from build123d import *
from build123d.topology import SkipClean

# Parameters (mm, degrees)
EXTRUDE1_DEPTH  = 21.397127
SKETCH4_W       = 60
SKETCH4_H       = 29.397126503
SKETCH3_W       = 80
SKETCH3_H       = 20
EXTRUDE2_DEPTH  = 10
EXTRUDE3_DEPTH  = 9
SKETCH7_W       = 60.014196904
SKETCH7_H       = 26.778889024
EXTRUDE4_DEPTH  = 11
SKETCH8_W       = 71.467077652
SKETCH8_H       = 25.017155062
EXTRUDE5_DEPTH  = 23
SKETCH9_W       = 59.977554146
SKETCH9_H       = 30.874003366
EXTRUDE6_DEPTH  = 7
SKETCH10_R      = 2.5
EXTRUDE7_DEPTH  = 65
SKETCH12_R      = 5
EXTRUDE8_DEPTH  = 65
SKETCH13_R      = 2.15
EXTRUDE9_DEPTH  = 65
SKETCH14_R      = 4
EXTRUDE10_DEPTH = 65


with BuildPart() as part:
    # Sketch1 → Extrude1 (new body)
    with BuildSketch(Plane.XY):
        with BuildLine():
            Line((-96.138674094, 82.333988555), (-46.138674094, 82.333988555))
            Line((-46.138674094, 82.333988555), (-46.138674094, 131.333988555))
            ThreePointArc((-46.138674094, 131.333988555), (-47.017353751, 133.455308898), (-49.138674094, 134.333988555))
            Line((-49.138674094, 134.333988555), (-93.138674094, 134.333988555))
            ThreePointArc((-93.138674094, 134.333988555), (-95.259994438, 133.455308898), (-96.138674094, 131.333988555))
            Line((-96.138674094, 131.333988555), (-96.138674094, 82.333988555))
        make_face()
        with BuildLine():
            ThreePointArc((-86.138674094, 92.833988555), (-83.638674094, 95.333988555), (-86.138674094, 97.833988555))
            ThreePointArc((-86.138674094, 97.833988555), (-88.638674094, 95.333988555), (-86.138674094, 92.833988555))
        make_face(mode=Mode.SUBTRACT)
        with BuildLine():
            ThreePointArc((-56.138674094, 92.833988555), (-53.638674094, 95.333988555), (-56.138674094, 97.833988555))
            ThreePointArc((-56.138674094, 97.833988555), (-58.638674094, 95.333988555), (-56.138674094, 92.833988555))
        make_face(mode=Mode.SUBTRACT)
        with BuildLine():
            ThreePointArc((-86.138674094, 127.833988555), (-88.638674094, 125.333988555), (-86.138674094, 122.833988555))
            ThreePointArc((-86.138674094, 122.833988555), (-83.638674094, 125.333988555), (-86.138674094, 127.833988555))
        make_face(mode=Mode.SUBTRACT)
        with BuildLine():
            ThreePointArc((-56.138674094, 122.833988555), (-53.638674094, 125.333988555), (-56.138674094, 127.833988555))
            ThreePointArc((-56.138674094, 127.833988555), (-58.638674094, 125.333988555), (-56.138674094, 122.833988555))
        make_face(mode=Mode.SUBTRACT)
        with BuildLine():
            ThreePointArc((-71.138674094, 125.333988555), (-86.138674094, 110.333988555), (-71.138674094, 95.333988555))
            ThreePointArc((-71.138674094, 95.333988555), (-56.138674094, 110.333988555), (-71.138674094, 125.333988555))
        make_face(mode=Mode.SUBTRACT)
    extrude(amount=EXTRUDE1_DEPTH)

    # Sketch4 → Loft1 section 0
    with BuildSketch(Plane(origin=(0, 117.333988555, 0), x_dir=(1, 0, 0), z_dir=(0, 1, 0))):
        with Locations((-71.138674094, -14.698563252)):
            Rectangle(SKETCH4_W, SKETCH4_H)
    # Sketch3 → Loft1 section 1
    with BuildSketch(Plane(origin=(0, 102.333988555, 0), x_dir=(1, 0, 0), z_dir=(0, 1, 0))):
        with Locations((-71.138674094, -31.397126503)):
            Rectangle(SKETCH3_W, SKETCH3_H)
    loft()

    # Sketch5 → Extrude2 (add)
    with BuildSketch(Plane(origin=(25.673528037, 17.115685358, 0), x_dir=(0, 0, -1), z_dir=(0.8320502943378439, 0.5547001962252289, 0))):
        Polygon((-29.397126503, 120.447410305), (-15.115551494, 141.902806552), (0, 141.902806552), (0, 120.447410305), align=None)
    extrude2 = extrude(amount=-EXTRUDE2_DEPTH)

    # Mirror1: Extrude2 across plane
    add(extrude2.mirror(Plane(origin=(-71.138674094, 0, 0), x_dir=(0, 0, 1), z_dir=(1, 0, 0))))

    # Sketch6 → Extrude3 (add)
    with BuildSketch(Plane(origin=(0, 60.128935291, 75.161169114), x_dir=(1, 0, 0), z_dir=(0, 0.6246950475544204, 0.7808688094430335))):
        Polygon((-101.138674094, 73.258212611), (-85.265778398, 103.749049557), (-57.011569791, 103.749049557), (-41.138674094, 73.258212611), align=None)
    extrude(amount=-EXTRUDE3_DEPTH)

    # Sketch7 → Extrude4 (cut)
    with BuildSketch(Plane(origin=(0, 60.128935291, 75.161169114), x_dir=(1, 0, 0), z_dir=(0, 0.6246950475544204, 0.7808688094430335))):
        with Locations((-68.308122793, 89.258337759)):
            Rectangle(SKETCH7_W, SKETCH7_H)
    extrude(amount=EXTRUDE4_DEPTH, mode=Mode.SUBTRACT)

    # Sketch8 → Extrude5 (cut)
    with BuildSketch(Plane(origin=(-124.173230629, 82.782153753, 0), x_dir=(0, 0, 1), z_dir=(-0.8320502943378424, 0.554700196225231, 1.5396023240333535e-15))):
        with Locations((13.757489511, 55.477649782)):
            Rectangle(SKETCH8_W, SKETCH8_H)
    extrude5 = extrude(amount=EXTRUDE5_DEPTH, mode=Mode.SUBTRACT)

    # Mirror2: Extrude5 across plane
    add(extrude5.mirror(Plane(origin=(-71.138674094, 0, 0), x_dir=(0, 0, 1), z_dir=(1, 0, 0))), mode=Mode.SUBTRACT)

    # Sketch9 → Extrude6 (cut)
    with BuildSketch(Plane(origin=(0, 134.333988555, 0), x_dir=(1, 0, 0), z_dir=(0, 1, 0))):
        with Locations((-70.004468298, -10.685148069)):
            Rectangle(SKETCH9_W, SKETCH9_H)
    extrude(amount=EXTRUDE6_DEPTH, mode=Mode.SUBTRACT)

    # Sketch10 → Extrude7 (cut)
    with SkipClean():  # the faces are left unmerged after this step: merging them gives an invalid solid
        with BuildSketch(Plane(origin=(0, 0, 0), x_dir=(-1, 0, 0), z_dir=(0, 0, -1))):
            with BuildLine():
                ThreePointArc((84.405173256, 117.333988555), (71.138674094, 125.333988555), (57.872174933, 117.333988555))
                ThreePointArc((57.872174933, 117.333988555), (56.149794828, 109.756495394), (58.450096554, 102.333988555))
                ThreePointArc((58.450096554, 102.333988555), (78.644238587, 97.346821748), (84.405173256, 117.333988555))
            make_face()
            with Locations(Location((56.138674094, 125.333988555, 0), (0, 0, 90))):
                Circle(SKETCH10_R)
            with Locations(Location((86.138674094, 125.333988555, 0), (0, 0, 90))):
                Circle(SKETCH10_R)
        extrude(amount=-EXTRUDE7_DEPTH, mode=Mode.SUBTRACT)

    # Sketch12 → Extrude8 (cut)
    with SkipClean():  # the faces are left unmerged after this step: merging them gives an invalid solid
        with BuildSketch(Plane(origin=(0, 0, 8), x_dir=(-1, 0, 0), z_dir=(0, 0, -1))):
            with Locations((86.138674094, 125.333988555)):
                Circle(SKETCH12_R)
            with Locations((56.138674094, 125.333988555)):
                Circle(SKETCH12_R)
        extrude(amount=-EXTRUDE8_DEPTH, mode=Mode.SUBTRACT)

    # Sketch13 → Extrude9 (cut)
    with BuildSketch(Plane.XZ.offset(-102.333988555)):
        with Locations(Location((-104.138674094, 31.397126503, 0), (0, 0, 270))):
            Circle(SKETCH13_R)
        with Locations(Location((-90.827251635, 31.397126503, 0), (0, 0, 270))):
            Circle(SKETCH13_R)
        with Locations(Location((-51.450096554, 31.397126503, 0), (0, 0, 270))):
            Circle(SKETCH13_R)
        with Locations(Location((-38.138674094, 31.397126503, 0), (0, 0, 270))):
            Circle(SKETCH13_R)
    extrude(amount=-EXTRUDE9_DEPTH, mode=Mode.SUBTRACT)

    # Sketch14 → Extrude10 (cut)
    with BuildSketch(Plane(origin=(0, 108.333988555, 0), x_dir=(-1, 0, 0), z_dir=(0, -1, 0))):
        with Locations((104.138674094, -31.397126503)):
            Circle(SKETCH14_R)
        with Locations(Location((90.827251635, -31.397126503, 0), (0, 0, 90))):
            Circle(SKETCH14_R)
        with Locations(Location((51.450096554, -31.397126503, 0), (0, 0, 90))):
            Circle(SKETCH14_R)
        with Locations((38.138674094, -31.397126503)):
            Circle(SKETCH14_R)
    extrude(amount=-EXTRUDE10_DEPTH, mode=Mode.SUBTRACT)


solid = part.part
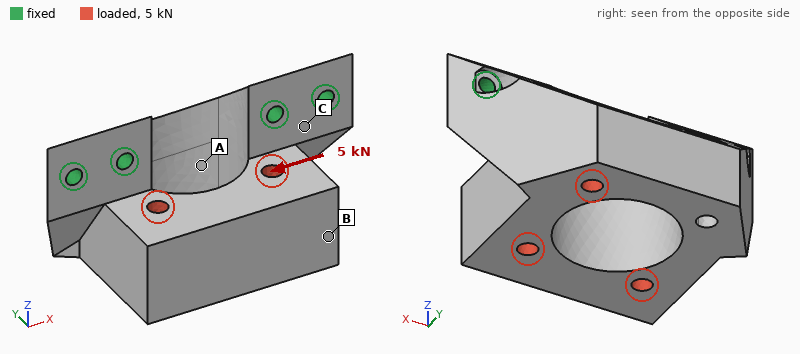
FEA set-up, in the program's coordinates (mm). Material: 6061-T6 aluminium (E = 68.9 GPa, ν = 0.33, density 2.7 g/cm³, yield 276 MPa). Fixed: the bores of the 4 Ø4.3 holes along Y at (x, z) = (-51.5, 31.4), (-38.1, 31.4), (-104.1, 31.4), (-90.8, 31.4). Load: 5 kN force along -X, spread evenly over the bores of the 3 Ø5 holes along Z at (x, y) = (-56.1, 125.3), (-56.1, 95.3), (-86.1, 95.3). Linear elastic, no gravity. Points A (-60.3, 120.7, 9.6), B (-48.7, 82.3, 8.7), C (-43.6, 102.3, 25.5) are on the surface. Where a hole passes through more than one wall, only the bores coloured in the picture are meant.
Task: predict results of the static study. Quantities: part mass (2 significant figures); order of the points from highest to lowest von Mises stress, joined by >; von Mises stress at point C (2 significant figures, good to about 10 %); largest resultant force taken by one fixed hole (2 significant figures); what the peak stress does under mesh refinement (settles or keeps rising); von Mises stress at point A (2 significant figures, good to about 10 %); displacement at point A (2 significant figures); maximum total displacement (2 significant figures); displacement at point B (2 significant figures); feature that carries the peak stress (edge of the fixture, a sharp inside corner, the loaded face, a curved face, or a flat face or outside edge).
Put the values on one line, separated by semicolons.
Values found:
130 g; C > A > B; 45 MPa; 2.4 kN; keeps rising; 20 MPa; 12 µm; 30 µm; 29 µm; edge of the fixture
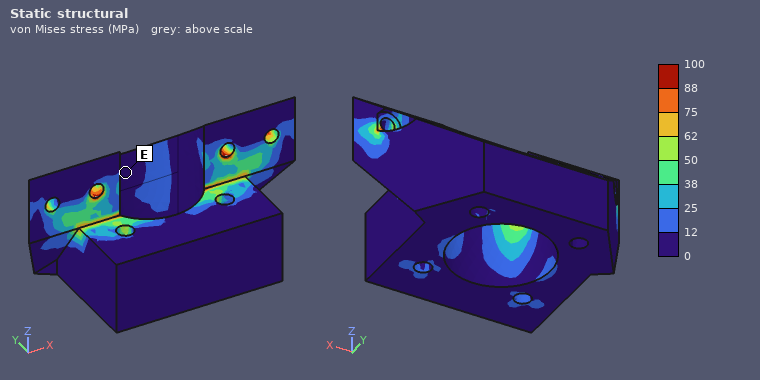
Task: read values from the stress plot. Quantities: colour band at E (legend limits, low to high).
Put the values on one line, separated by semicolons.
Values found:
0 to 12 MPa
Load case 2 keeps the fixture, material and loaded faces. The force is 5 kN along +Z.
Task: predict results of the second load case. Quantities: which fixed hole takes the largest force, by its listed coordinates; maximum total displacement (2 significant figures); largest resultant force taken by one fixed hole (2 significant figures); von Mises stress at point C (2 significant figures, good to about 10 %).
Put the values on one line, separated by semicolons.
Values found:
(-51.5, 31.4); 85 µm; 2.0 kN; 34 MPa
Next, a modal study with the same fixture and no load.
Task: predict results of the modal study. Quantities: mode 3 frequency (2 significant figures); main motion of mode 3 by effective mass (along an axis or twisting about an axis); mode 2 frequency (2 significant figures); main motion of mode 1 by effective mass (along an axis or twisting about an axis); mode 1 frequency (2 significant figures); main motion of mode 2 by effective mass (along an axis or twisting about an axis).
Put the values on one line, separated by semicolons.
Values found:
9600 Hz; along X; 7400 Hz; along Y; 2500 Hz; along X
